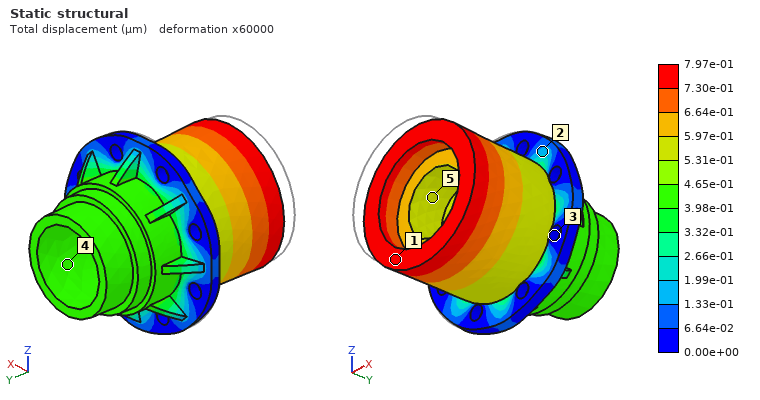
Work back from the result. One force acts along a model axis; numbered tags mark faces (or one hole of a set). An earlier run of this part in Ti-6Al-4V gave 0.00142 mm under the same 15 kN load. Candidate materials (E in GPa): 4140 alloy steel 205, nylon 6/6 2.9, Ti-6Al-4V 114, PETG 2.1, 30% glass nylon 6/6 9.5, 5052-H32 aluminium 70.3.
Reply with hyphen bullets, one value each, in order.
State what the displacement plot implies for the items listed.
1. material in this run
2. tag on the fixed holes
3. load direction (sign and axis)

- 4140 alloy steel
- 3
- +Y
